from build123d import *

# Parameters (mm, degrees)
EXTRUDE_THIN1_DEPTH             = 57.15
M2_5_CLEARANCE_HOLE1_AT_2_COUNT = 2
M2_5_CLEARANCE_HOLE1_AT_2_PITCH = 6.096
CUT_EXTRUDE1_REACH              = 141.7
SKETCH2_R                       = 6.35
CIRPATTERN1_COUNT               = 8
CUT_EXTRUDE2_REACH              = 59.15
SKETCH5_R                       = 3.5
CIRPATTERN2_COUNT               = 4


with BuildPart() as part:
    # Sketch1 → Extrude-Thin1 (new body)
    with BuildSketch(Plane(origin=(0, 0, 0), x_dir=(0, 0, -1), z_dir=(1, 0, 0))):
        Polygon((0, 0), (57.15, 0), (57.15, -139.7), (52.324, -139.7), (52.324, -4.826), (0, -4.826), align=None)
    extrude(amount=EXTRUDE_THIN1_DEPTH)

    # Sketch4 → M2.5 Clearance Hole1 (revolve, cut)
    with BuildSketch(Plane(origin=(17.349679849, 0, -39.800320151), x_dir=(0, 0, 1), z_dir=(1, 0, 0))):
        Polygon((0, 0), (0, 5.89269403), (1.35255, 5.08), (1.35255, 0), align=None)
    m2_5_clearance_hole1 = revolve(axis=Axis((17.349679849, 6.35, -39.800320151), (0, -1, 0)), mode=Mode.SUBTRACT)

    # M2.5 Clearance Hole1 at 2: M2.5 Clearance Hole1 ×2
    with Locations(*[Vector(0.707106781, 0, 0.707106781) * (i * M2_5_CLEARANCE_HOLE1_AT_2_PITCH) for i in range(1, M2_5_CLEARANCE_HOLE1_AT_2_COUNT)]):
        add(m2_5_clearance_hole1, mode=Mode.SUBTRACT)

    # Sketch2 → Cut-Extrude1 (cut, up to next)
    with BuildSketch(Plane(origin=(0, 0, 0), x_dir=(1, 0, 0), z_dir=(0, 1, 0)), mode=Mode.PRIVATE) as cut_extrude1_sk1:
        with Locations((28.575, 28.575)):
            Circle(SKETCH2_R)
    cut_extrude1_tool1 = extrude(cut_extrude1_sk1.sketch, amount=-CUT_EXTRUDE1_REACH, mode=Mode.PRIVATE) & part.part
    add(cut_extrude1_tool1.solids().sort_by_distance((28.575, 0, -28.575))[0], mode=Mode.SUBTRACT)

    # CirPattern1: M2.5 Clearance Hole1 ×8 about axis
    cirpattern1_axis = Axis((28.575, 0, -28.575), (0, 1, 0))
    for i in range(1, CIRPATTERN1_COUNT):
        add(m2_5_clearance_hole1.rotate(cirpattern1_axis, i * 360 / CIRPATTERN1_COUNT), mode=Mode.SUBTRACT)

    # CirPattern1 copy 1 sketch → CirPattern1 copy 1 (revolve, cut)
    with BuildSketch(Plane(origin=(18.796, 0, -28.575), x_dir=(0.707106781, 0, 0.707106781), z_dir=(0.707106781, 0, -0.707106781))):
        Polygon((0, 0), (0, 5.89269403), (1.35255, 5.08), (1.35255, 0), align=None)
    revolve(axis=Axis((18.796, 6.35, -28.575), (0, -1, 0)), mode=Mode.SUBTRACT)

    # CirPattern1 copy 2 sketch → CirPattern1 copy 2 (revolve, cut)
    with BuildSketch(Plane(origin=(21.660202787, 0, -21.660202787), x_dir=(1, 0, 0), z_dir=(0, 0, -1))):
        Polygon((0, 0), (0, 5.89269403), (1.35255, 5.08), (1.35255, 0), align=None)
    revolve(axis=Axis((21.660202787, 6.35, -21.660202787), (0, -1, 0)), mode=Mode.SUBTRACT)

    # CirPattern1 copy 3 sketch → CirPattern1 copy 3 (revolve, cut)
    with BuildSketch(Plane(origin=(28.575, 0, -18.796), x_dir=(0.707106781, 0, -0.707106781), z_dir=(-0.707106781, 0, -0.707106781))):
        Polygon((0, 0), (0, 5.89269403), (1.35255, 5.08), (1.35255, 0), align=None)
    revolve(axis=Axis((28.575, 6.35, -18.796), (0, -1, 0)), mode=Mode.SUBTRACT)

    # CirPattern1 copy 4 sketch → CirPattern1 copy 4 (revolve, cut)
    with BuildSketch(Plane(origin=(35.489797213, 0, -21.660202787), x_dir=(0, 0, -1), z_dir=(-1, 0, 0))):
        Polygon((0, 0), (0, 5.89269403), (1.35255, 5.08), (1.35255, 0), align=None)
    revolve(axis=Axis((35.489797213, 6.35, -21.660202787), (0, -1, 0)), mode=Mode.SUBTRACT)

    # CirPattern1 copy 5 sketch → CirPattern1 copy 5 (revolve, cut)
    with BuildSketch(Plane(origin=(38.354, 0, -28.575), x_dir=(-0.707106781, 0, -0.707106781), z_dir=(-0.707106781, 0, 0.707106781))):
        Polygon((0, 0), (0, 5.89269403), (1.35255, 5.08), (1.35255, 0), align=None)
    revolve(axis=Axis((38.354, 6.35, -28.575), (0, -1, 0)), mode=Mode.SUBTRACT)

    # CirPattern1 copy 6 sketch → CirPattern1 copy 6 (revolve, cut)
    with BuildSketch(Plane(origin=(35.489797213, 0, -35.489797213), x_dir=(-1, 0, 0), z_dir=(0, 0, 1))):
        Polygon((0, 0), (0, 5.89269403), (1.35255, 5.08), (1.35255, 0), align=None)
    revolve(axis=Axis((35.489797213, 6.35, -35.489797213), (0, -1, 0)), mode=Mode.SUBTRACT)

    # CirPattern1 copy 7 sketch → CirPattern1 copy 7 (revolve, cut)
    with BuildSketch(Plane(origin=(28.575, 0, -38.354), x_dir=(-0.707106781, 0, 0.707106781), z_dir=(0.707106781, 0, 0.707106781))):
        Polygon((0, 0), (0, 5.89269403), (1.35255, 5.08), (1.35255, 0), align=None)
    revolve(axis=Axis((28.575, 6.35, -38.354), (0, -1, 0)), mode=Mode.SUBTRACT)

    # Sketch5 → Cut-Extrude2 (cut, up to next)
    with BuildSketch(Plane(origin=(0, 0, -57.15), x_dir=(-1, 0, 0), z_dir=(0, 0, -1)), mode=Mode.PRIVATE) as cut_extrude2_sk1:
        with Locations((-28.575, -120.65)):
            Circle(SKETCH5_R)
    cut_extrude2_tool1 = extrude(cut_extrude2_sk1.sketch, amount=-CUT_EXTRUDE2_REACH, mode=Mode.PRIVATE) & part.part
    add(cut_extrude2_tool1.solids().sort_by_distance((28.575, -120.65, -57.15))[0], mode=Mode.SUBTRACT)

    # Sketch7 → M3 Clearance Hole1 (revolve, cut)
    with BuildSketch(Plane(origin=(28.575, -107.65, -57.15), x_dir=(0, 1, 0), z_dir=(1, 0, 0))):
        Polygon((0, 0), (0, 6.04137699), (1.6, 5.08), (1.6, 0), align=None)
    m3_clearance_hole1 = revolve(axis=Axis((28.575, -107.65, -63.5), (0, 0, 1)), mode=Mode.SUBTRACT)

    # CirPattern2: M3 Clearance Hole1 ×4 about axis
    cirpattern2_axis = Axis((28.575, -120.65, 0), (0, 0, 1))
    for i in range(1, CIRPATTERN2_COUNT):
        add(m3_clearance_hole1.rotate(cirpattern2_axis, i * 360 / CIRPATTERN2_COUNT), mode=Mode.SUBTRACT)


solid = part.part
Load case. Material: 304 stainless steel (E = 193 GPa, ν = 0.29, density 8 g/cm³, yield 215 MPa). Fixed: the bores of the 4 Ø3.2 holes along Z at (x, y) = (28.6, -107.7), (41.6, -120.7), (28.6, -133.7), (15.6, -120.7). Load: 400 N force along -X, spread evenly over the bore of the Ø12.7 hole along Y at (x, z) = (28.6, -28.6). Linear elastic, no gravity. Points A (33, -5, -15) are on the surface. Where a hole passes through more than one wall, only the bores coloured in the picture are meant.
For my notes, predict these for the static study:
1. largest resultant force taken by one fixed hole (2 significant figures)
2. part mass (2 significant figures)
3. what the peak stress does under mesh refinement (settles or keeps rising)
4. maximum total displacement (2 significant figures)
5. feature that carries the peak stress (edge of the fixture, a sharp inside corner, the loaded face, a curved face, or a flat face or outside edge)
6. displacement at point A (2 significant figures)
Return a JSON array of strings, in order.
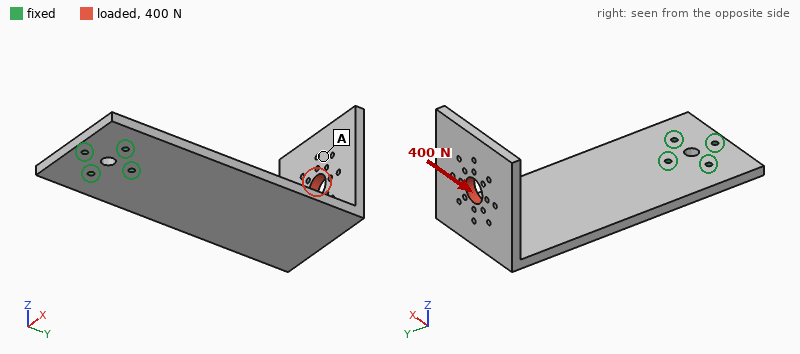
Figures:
["1.1 kN", "410 g", "keeps rising", "0.44 mm", "edge of the fixture", "0.30 mm"]
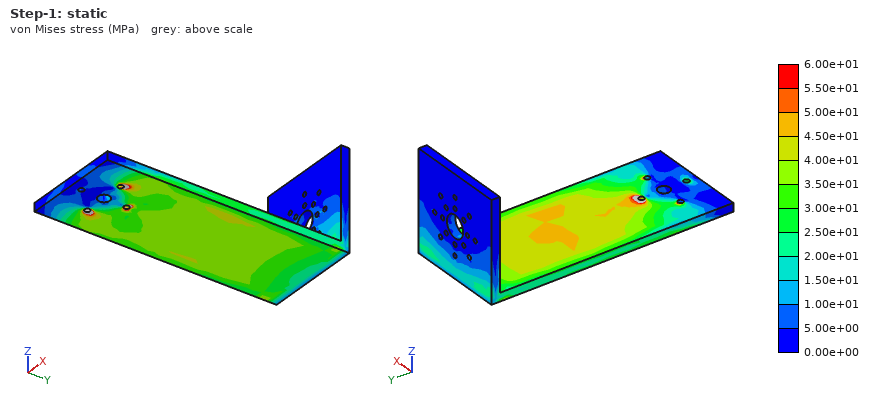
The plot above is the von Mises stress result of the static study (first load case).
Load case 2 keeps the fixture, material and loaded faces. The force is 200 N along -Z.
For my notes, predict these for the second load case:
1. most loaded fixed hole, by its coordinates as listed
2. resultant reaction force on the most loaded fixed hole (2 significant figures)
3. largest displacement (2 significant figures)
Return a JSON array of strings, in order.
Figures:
["(28.6, -107.7)", "1.1 kN", "1.0 mm"]
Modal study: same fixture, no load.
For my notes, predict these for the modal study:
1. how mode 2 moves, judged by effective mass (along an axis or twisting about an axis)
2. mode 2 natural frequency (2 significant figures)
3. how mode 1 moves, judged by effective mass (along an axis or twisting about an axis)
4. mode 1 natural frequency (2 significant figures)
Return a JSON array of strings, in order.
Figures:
["along X", "470 Hz", "along Z", "180 Hz"]
